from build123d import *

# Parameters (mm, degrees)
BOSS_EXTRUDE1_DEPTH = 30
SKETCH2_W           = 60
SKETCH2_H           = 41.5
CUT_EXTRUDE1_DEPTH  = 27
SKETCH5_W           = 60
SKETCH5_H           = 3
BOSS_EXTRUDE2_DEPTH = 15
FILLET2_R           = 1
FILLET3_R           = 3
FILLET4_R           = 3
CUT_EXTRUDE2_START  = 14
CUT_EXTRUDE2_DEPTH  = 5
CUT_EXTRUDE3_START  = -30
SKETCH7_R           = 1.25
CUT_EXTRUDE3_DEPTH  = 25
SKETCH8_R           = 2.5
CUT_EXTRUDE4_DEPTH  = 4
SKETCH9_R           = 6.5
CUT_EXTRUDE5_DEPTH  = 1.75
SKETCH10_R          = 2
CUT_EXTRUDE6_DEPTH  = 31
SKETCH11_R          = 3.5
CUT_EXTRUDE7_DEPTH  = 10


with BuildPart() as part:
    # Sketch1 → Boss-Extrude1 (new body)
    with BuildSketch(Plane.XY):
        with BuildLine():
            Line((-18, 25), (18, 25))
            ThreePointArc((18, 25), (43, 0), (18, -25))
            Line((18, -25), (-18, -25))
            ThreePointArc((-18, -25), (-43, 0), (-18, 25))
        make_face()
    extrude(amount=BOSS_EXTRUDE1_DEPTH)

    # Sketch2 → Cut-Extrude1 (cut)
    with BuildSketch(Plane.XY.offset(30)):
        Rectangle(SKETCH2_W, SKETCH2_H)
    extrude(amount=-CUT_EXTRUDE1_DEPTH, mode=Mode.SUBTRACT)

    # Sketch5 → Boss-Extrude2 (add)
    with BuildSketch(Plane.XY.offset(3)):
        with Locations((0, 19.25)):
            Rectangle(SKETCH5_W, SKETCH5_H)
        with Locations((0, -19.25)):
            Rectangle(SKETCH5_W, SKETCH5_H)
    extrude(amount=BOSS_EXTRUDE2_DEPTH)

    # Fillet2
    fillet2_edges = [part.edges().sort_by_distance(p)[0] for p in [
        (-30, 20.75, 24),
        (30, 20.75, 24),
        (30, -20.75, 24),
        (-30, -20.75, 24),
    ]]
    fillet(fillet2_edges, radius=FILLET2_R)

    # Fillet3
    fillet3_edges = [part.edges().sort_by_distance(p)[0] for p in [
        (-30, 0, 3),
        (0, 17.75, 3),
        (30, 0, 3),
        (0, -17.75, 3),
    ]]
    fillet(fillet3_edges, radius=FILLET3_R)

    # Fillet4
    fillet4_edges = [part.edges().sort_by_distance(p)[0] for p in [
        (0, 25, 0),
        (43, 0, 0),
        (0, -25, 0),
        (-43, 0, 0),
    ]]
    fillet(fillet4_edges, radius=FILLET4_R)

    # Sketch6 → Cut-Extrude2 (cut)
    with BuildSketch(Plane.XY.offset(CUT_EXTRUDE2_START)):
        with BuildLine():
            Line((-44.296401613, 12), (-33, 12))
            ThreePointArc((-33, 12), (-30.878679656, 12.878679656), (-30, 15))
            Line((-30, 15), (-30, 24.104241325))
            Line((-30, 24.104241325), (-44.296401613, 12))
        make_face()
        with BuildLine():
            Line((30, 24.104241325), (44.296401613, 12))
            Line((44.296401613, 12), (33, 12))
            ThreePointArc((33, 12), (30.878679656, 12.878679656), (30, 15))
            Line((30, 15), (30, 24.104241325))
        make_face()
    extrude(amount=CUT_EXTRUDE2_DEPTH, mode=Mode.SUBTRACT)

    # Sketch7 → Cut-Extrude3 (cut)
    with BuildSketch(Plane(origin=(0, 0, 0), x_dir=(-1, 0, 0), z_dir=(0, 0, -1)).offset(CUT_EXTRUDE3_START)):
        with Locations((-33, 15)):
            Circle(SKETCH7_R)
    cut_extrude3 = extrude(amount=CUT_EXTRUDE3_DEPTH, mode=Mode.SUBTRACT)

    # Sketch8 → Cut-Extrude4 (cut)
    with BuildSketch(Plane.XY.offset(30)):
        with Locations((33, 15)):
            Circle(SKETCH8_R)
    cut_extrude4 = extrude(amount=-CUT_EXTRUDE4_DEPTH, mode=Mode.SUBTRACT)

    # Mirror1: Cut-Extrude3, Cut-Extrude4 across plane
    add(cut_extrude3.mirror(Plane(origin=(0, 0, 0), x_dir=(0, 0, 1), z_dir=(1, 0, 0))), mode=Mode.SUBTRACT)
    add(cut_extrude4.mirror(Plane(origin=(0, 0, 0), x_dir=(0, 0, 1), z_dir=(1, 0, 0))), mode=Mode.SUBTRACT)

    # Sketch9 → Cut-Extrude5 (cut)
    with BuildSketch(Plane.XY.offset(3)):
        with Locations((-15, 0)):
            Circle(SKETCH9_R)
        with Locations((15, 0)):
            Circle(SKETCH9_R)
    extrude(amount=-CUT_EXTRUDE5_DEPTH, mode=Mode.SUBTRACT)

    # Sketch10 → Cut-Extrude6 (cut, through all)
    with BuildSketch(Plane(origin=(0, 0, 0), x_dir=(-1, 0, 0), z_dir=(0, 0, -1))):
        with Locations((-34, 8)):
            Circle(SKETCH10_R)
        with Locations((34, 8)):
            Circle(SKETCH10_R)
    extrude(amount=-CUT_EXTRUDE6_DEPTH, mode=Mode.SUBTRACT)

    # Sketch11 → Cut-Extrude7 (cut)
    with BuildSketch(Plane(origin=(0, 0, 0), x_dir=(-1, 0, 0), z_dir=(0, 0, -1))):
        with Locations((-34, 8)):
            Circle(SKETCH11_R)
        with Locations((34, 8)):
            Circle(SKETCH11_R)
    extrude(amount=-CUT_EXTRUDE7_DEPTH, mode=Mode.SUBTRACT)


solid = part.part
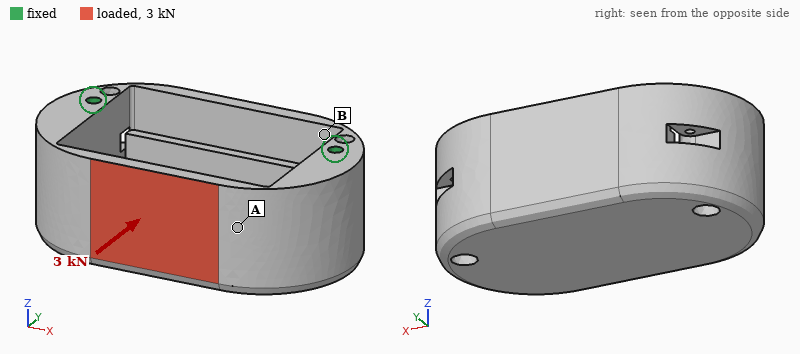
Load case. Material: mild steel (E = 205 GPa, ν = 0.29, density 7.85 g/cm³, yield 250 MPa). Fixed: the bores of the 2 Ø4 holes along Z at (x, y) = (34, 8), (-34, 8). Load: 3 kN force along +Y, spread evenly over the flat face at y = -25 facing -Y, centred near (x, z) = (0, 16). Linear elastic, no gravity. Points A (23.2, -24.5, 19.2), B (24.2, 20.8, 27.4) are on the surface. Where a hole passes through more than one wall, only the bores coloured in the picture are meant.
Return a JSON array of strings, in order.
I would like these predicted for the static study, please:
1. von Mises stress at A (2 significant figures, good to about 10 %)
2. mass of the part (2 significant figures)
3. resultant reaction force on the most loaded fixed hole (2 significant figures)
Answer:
["68 MPa", "380 g", "1.7 kN"]
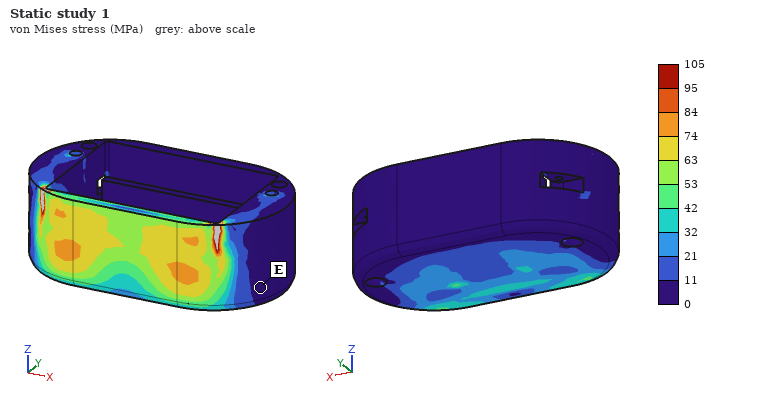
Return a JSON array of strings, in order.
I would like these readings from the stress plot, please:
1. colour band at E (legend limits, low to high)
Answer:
["0 to 11 MPa"]
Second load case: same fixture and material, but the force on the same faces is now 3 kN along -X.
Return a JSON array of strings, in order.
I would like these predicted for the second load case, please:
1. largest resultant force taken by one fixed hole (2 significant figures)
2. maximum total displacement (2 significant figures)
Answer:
["1.9 kN", "13 µm"]
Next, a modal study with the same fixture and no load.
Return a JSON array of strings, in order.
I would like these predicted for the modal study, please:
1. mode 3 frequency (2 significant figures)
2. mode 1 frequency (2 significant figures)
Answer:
["7100 Hz", "6400 Hz"]
